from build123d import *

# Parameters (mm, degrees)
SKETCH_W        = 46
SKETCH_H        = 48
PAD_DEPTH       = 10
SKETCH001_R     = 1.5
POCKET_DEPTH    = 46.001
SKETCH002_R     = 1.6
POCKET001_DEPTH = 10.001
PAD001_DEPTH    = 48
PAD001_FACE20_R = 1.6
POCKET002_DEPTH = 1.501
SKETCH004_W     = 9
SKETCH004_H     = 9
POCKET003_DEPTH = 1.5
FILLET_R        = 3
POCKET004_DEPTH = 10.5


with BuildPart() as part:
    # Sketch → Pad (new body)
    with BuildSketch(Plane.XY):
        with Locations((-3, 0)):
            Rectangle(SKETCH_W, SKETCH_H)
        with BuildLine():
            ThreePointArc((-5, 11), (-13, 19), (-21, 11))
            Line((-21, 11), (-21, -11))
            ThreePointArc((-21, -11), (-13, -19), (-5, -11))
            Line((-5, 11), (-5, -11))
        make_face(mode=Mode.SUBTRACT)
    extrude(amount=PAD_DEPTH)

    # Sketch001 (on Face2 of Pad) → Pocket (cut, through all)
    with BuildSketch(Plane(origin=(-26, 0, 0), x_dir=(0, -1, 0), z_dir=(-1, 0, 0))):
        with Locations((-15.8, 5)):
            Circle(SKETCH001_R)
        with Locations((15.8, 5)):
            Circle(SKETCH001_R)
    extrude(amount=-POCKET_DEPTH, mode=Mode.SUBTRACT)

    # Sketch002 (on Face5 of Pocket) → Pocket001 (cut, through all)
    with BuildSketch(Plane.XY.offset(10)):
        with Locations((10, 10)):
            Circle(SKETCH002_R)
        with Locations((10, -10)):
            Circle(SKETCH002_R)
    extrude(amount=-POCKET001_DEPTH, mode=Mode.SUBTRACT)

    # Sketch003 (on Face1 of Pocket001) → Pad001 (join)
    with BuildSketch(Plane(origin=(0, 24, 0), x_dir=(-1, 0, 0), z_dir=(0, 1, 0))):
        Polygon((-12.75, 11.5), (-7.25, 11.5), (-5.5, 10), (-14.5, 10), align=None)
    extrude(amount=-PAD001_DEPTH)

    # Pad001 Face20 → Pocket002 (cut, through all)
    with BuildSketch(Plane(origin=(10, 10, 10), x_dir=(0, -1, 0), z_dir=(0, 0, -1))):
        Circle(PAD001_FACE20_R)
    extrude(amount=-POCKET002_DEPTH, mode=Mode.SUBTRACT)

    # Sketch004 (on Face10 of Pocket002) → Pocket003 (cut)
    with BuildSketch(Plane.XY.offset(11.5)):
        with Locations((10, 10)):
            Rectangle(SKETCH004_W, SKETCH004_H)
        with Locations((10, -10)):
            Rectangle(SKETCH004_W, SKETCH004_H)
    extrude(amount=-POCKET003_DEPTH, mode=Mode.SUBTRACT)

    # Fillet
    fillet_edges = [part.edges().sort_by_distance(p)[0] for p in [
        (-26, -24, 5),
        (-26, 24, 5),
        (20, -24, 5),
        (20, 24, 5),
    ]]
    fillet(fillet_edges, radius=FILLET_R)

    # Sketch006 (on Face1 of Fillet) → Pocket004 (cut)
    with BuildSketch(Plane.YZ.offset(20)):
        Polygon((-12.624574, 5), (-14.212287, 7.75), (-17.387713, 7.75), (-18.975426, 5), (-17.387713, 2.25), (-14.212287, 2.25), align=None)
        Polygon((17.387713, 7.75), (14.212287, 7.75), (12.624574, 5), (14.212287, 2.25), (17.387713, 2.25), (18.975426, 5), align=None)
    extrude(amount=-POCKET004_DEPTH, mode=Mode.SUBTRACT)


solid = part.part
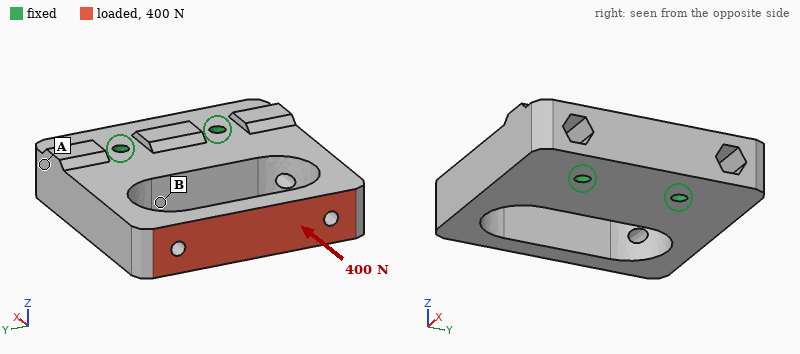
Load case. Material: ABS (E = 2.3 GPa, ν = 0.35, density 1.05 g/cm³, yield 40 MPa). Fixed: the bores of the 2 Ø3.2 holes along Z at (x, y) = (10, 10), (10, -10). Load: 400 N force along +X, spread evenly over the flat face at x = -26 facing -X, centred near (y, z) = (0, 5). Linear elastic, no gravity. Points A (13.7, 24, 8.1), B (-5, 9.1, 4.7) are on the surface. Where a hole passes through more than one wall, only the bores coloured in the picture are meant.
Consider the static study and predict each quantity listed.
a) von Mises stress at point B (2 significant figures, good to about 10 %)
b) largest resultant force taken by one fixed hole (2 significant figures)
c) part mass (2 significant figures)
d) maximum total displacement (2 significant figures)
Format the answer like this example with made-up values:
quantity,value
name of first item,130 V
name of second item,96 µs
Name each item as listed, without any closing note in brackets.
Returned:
quantity,value
von Mises stress at point B,5.2 MPa
largest resultant force taken by one fixed hole,210 N
part mass,17 g
maximum total displacement,0.46 mm
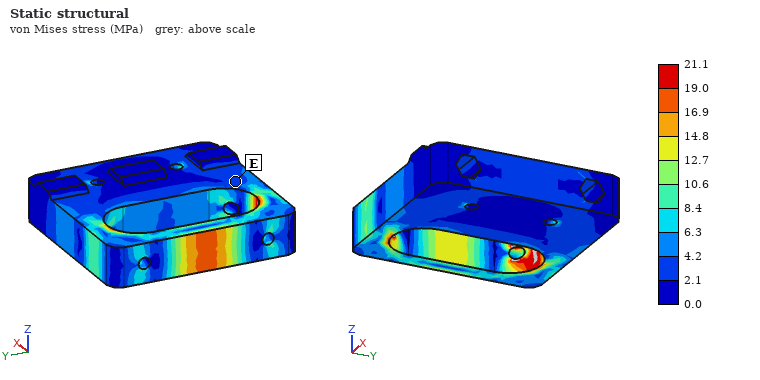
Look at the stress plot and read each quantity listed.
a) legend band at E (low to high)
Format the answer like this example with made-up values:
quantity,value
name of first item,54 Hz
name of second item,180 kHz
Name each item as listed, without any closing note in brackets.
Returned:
quantity,value
legend band at E,2.1 to 4.2 MPa
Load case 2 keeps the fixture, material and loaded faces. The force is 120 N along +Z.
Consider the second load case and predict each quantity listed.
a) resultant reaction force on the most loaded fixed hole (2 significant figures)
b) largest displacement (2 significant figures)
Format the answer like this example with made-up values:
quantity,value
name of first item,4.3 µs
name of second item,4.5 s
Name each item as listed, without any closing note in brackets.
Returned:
quantity,value
resultant reaction force on the most loaded fixed hole,60 N
largest displacement,0.70 mm
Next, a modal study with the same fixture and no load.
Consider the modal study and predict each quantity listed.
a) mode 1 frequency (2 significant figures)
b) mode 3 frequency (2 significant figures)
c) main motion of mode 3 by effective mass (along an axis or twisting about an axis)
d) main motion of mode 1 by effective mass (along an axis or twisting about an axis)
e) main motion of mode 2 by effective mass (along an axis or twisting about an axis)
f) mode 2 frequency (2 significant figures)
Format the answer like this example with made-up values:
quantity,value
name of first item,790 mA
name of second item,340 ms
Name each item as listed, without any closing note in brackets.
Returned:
quantity,value
mode 1 frequency,1400 Hz
mode 3 frequency,2300 Hz
main motion of mode 3 by effective mass,twisting about X
main motion of mode 1 by effective mass,along Z
main motion of mode 2 by effective mass,along Y
mode 2 frequency,2100 Hz
